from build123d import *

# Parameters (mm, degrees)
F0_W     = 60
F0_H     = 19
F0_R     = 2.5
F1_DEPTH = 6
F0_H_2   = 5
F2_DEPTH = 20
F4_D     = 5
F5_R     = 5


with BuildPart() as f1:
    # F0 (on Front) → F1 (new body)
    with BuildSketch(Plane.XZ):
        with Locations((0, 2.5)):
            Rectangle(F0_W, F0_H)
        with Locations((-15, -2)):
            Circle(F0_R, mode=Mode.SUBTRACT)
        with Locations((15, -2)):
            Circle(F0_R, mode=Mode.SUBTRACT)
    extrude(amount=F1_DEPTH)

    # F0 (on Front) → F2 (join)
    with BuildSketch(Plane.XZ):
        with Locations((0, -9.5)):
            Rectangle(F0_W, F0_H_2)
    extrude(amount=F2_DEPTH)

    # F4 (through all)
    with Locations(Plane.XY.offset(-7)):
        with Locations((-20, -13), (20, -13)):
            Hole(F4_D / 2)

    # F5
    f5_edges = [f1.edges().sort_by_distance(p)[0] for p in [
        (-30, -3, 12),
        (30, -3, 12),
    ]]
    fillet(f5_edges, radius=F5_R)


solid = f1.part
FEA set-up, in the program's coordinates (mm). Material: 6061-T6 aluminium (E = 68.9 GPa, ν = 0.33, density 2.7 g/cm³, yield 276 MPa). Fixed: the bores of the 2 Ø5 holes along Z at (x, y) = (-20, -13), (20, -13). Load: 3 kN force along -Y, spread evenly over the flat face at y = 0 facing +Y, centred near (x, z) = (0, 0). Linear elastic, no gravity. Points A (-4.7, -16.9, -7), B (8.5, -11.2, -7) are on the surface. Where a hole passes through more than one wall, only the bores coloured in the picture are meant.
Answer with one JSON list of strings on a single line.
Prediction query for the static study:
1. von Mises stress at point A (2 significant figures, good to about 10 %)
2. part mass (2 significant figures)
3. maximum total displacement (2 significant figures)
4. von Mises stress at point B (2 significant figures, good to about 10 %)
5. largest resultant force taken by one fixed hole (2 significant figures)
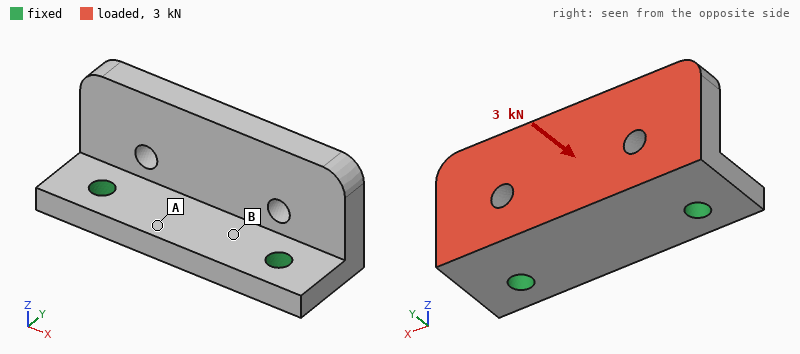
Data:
["31 MPa", "33 g", "0.20 mm", "66 MPa", "1.5 kN"]
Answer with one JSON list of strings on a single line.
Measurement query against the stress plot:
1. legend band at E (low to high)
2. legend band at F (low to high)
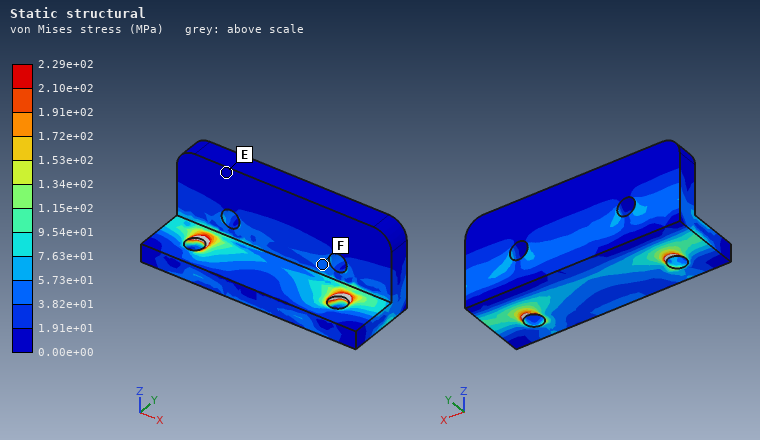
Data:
["0.00e+00 to 1.91e+01 MPa", "3.82e+01 to 5.73e+01 MPa"]
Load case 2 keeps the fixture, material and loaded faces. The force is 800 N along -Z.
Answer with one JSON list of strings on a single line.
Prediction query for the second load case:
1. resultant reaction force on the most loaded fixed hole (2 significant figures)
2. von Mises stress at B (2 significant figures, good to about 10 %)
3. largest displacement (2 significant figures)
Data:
["400 N", "13 MPa", "46 µm"]
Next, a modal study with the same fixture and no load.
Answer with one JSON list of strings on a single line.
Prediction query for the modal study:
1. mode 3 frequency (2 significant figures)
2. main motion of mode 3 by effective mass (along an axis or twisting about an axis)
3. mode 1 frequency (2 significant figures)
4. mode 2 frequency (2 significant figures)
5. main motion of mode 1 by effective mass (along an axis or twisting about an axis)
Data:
["14 kHz", "along Z", "4700 Hz", "8200 Hz", "along Y"]
